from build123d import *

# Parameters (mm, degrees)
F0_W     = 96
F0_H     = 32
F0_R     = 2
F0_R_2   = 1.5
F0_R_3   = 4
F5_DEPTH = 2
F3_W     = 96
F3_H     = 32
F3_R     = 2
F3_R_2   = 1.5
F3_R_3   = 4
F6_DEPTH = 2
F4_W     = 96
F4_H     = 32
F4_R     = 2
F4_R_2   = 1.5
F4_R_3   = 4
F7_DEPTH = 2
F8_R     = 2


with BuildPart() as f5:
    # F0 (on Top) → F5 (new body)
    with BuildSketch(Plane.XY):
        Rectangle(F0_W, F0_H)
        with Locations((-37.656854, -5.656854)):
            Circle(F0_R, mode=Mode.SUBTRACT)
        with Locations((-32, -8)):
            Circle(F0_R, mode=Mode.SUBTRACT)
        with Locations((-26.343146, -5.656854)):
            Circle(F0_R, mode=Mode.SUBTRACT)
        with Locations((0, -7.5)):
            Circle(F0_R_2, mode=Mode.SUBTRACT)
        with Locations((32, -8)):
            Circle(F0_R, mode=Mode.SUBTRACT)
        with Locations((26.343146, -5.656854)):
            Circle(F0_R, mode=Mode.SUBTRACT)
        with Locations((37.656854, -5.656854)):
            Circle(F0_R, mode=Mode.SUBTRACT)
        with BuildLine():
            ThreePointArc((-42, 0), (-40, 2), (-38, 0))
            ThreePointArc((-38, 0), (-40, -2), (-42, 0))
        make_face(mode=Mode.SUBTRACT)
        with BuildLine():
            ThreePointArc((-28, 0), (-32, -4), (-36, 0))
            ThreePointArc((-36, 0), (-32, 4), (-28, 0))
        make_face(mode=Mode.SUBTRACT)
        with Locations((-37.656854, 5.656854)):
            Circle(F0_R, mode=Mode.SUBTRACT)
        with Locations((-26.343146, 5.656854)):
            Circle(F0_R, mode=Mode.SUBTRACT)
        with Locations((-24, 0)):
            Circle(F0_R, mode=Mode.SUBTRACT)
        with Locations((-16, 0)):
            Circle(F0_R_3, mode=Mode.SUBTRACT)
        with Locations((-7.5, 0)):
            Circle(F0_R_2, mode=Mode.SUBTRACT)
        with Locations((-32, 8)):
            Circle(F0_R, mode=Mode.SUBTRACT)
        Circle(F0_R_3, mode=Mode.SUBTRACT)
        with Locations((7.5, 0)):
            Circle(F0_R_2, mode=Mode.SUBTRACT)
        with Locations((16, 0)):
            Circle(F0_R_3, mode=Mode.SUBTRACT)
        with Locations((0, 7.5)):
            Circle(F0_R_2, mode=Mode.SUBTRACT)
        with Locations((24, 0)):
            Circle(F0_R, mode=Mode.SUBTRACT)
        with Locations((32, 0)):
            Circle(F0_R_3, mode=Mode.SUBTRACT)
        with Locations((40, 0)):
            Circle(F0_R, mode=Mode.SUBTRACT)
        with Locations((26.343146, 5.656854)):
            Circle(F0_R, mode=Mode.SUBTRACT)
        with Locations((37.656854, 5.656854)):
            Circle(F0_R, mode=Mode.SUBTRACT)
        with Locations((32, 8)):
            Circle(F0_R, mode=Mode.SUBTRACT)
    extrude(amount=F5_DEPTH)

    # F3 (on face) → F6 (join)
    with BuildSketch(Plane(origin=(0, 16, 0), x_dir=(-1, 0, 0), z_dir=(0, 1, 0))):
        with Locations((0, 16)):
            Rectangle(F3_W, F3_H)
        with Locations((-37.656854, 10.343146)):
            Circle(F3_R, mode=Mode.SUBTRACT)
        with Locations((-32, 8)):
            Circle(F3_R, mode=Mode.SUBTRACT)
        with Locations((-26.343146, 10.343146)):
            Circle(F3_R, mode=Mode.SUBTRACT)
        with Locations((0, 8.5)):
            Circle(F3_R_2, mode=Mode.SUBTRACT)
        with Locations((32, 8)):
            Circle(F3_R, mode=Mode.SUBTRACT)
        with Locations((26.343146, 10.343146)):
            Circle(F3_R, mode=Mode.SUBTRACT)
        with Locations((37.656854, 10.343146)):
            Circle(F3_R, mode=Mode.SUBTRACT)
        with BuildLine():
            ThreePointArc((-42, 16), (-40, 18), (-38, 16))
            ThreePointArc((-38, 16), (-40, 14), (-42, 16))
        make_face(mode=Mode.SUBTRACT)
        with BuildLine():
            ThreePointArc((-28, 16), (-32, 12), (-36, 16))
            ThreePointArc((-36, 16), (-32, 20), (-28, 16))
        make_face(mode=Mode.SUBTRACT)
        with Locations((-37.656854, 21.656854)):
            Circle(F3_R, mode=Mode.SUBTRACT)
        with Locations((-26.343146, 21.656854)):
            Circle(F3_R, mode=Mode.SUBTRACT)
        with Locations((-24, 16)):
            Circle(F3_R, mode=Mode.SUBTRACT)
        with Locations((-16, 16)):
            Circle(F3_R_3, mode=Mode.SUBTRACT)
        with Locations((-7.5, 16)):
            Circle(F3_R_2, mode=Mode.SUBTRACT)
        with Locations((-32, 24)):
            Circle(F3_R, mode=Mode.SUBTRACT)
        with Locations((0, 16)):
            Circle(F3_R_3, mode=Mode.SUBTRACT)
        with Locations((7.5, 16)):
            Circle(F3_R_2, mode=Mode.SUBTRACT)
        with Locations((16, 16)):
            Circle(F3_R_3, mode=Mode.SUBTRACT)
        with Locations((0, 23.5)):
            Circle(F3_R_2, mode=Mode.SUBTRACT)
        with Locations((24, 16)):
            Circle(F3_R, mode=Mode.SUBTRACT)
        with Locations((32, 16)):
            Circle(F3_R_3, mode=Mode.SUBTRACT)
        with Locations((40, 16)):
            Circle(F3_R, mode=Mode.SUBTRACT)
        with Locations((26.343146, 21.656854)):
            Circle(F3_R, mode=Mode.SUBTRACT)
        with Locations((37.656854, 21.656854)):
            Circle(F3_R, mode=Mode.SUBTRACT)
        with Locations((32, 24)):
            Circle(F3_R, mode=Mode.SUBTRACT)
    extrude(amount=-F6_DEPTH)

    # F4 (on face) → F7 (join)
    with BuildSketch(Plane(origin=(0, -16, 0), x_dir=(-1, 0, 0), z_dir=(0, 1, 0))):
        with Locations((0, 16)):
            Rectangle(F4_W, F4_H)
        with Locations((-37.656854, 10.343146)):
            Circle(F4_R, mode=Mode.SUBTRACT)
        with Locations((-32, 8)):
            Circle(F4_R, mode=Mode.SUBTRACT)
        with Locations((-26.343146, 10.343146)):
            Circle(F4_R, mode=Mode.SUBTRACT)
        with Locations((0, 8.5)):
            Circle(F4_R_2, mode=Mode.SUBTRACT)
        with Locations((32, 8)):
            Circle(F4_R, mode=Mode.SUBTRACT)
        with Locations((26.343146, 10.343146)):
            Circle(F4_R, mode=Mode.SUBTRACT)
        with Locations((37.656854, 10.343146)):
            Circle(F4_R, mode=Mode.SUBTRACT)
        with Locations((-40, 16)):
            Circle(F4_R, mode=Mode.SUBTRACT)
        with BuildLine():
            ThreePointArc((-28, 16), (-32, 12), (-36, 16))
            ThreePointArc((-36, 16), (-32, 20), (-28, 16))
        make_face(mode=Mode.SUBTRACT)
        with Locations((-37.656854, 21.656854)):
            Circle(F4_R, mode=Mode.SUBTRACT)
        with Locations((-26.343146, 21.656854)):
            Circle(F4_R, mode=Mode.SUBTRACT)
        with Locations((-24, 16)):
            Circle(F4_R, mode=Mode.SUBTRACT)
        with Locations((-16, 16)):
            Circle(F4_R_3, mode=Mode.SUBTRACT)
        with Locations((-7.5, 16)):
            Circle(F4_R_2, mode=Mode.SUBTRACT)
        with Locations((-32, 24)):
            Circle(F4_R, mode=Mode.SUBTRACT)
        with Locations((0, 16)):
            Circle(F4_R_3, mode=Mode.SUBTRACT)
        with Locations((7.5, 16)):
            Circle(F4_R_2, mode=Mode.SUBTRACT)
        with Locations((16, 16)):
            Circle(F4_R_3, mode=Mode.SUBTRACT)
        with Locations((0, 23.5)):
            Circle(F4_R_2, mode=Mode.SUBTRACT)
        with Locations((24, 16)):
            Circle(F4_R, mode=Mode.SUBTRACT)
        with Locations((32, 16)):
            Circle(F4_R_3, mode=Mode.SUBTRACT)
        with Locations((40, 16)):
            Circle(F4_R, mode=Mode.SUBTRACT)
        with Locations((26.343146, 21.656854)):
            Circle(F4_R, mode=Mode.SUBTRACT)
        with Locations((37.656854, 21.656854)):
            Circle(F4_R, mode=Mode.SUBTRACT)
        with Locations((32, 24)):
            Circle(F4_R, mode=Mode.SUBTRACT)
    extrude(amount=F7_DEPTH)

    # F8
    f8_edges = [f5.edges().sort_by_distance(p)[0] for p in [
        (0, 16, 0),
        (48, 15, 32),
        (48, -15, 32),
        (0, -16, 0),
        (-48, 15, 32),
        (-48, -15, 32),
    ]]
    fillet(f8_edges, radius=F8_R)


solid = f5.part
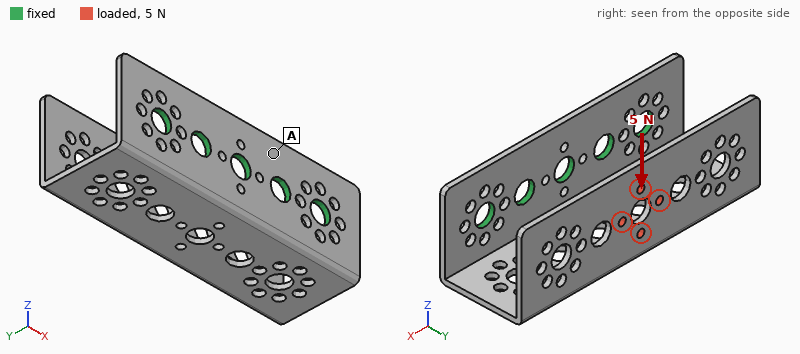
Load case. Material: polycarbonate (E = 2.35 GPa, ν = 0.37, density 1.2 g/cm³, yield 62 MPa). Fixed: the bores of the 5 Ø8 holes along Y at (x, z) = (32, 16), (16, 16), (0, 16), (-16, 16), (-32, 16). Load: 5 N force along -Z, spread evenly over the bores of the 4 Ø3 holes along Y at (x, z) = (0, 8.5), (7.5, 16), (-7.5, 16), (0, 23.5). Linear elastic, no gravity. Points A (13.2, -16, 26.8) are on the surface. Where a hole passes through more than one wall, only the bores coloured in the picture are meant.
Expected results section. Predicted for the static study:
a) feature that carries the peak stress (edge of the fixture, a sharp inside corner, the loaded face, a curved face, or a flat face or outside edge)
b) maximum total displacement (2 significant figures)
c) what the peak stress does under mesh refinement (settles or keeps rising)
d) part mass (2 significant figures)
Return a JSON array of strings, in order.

["a sharp inside corner", "1.2 mm", "keeps rising", "18 g"]
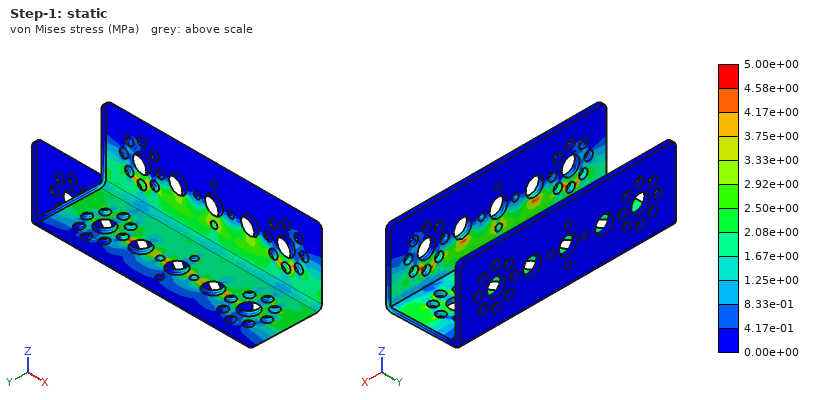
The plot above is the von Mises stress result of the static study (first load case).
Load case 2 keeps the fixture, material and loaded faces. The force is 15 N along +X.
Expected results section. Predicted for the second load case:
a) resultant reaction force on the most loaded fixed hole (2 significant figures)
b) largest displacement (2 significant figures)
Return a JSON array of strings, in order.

["5.4 N", "1.2 mm"]
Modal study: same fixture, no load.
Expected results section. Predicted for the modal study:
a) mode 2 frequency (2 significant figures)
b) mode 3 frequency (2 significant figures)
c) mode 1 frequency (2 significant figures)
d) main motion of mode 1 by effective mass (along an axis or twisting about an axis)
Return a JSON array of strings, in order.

["200 Hz", "330 Hz", "120 Hz", "along Z"]
